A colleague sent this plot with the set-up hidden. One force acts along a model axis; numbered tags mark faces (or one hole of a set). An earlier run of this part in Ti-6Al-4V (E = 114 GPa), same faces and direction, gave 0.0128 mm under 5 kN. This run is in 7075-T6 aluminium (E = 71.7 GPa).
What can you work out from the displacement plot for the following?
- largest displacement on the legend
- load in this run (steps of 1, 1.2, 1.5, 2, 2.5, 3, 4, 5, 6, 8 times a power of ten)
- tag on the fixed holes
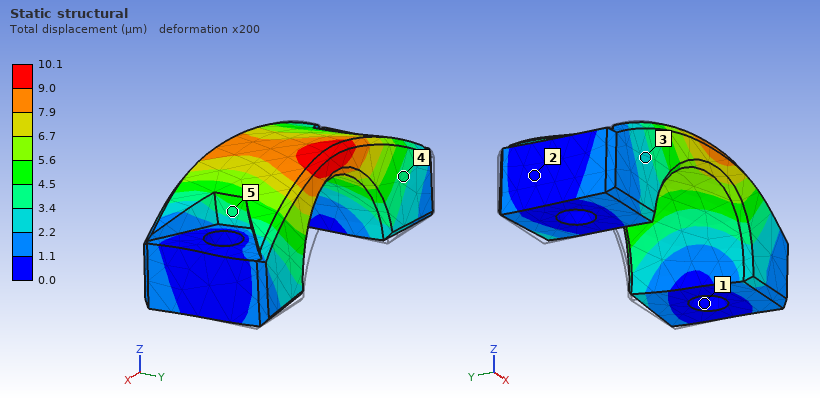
10.1 µm
2.5 kN
1
